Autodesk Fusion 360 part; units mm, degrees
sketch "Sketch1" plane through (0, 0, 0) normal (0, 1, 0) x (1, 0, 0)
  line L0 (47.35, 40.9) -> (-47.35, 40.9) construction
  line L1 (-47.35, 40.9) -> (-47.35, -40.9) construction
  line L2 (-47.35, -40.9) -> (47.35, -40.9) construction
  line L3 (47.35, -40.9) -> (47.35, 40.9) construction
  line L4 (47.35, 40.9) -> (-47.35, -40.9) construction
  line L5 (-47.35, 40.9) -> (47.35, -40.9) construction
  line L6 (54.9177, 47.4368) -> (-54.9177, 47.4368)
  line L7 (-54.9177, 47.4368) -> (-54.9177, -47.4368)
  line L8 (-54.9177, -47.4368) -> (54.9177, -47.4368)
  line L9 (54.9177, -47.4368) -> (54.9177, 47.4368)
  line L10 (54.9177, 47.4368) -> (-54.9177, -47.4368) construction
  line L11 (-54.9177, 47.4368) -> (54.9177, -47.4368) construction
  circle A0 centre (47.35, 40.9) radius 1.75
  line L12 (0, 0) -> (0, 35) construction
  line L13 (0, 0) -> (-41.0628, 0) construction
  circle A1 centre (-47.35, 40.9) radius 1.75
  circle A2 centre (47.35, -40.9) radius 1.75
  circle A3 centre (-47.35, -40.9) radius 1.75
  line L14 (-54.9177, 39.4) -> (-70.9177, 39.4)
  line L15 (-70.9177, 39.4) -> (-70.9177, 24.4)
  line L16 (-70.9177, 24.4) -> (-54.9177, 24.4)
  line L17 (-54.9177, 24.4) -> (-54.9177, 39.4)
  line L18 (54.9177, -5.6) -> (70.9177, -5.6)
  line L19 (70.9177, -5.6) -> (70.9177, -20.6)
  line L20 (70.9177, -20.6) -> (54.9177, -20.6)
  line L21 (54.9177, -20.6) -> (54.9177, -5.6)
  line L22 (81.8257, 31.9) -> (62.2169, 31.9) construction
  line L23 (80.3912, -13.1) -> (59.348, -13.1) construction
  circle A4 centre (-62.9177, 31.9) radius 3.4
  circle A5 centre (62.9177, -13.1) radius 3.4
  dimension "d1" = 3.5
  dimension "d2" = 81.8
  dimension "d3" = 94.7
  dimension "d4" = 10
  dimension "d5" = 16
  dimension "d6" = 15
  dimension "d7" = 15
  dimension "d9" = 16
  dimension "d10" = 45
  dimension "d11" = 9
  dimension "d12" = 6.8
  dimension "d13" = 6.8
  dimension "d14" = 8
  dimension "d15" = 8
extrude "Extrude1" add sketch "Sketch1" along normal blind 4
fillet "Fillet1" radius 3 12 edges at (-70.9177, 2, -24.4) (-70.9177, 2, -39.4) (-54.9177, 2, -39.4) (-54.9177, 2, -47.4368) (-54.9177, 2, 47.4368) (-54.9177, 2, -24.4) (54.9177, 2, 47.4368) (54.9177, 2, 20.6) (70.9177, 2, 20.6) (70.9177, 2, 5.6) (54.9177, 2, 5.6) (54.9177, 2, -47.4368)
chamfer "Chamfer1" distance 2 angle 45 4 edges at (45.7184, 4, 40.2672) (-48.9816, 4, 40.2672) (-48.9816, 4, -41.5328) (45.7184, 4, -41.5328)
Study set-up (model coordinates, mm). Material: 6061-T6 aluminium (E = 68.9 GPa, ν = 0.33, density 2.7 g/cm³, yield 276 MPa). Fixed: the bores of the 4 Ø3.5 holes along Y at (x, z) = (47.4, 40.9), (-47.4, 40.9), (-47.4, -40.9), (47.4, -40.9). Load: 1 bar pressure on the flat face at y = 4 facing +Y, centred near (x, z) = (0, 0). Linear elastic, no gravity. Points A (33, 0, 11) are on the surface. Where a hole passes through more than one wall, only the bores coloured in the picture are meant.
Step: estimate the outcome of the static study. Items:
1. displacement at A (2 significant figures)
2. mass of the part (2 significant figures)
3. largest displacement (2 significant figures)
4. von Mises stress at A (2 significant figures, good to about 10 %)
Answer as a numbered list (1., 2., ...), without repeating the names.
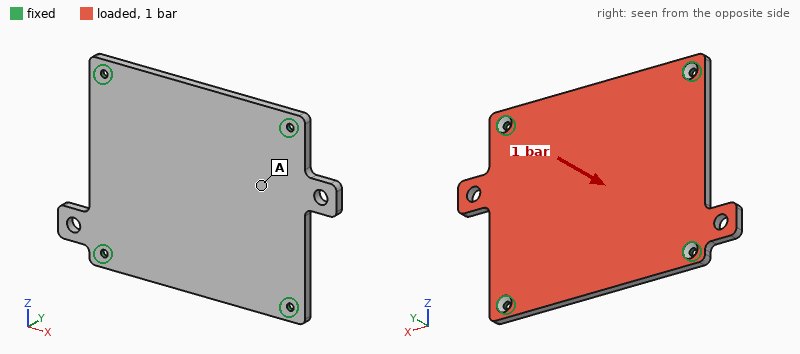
1. 0.11 mm
2. 120 g
3. 0.16 mm
4. 14 MPa
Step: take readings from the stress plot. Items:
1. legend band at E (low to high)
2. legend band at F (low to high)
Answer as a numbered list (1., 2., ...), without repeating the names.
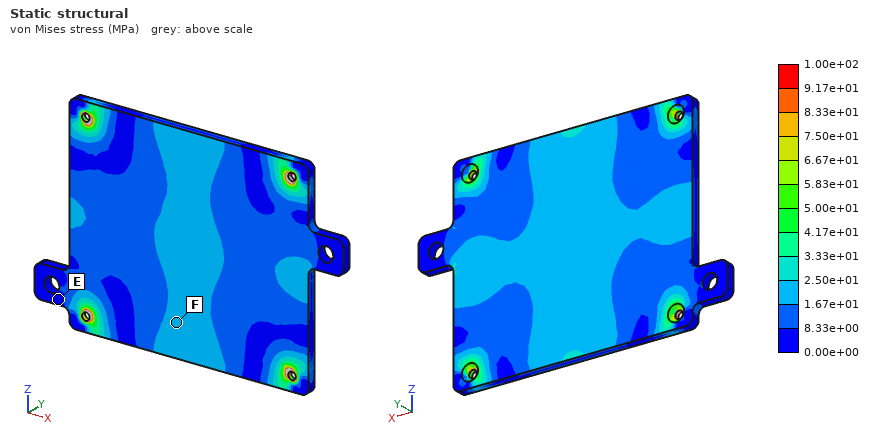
1. 0.00e+00 to 8.33e+00 MPa
2. 1.67e+01 to 2.50e+01 MPa
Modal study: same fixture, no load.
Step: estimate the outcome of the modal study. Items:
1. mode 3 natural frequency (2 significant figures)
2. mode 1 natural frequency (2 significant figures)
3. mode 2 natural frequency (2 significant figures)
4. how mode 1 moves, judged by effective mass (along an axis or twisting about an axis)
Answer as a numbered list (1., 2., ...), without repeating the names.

1. 2400 Hz
2. 1400 Hz
3. 2400 Hz
4. along Y
